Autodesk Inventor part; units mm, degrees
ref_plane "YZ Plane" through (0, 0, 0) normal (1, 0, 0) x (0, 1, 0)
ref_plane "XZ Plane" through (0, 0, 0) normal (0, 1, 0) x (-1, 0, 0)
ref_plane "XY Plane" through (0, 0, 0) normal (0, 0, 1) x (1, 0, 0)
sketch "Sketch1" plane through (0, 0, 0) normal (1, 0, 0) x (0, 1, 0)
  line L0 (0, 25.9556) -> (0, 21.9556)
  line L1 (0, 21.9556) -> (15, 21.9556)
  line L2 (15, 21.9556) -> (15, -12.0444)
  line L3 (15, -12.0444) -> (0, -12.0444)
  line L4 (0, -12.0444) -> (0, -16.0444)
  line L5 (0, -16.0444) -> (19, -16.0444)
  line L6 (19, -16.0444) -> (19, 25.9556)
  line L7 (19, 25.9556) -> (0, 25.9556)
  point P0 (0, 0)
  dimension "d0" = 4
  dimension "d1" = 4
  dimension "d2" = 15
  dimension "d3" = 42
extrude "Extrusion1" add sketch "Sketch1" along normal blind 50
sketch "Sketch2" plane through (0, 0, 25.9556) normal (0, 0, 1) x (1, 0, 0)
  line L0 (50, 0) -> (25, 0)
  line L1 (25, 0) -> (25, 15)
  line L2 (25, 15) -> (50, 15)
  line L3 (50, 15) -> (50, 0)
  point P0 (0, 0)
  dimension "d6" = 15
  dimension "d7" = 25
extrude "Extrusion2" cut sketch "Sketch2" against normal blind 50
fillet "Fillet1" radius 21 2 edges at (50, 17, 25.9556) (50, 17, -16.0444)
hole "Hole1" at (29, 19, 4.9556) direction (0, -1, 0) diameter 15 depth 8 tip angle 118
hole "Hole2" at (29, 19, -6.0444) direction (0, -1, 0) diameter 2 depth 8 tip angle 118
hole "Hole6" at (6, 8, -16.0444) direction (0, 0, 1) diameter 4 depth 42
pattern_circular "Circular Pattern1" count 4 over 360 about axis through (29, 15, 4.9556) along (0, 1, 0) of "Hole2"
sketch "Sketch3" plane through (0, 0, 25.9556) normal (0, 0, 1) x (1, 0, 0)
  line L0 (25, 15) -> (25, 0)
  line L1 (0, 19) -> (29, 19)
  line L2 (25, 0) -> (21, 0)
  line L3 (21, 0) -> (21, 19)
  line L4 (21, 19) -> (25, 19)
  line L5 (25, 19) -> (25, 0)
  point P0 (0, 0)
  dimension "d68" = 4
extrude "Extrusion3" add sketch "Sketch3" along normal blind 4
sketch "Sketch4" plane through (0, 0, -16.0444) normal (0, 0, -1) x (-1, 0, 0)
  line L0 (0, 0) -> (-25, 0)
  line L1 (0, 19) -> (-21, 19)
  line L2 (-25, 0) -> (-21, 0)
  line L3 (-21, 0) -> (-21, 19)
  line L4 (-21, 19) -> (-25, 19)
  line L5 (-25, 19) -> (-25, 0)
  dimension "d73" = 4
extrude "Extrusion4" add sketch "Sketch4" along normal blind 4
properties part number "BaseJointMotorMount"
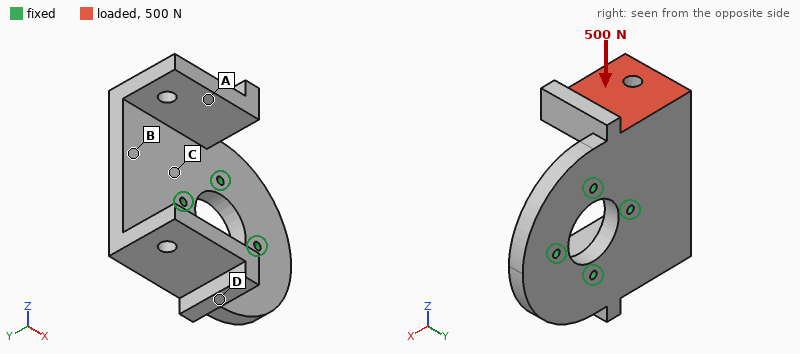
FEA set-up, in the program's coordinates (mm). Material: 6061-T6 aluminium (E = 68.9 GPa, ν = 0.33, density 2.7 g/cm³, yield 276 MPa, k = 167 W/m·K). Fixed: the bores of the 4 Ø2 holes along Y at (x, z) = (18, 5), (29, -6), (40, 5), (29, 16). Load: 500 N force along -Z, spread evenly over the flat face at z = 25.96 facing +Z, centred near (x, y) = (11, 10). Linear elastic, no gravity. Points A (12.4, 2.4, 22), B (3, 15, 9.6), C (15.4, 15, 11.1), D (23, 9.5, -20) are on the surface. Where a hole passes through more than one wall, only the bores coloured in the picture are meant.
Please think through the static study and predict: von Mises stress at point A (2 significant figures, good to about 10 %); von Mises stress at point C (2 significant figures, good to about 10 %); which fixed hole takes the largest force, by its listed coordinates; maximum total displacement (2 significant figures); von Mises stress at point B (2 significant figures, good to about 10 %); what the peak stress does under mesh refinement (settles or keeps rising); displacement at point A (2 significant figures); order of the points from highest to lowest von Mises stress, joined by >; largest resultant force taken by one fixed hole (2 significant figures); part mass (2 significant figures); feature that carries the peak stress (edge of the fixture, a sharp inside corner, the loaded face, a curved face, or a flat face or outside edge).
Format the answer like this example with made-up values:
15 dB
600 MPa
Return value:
13 MPa
34 MPa
(18, 5)
0.12 mm
26 MPa
keeps rising
0.082 mm
C > B > A > D
480 N
28 g
edge of the fixture
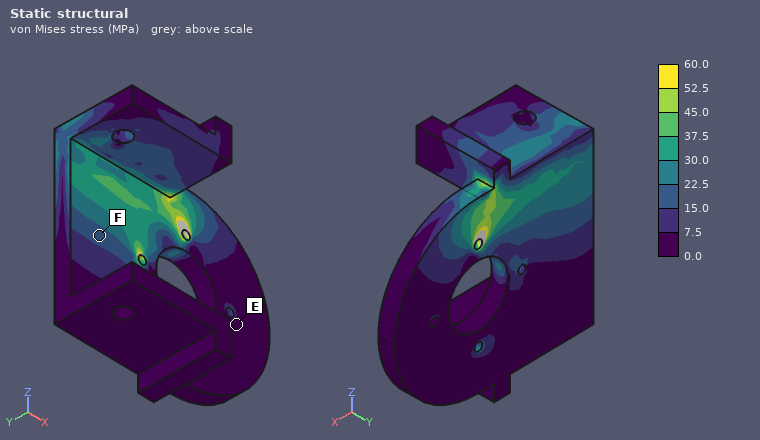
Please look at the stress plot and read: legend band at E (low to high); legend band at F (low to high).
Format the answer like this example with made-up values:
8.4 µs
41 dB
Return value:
0.0 to 7.5 MPa
15.0 to 22.5 MPa
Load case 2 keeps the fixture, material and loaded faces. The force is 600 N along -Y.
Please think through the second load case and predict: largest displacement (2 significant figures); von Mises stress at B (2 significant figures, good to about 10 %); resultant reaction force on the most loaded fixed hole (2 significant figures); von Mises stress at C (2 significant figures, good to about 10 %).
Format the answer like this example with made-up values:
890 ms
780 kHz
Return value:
0.30 mm
58 MPa
450 N
76 MPa
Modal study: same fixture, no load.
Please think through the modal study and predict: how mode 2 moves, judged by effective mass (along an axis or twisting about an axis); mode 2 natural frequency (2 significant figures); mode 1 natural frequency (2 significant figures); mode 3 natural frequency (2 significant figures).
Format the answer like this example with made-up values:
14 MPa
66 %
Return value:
along Y
3800 Hz
3500 Hz
6700 Hz
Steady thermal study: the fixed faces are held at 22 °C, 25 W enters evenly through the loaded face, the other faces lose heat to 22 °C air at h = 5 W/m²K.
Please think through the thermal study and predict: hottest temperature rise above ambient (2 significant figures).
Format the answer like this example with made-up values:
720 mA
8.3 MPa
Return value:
34 K
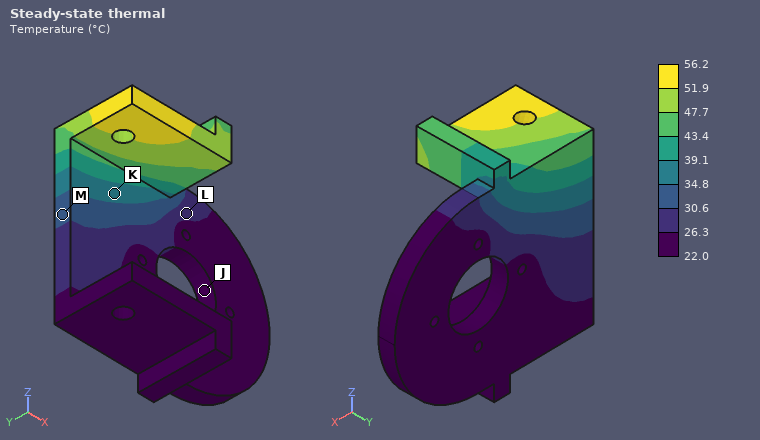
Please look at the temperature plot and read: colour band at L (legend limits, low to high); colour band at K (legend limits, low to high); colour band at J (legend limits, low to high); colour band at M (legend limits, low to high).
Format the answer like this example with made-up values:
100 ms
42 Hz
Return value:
26.3 to 30.6 °C
34.8 to 39.1 °C
22.0 to 26.3 °C
30.6 to 34.8 °C
